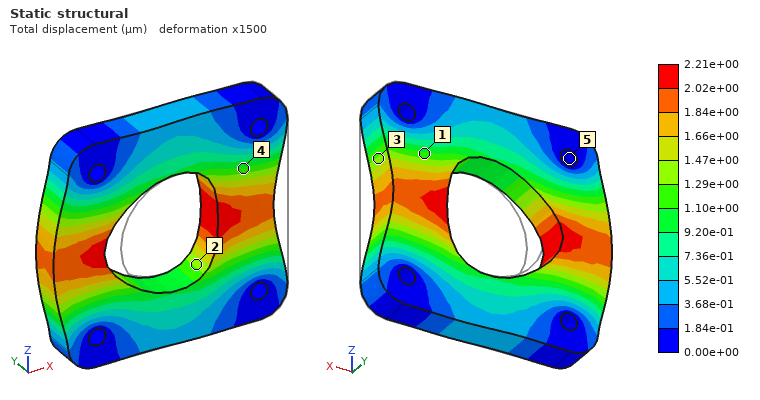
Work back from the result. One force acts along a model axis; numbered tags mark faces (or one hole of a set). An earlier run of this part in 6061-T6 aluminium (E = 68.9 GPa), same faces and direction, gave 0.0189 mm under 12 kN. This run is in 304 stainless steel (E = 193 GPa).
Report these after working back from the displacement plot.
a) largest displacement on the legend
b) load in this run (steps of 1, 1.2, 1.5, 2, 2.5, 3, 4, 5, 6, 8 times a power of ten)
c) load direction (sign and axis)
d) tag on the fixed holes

2.21e+00 µm
4 kN
-X
5
